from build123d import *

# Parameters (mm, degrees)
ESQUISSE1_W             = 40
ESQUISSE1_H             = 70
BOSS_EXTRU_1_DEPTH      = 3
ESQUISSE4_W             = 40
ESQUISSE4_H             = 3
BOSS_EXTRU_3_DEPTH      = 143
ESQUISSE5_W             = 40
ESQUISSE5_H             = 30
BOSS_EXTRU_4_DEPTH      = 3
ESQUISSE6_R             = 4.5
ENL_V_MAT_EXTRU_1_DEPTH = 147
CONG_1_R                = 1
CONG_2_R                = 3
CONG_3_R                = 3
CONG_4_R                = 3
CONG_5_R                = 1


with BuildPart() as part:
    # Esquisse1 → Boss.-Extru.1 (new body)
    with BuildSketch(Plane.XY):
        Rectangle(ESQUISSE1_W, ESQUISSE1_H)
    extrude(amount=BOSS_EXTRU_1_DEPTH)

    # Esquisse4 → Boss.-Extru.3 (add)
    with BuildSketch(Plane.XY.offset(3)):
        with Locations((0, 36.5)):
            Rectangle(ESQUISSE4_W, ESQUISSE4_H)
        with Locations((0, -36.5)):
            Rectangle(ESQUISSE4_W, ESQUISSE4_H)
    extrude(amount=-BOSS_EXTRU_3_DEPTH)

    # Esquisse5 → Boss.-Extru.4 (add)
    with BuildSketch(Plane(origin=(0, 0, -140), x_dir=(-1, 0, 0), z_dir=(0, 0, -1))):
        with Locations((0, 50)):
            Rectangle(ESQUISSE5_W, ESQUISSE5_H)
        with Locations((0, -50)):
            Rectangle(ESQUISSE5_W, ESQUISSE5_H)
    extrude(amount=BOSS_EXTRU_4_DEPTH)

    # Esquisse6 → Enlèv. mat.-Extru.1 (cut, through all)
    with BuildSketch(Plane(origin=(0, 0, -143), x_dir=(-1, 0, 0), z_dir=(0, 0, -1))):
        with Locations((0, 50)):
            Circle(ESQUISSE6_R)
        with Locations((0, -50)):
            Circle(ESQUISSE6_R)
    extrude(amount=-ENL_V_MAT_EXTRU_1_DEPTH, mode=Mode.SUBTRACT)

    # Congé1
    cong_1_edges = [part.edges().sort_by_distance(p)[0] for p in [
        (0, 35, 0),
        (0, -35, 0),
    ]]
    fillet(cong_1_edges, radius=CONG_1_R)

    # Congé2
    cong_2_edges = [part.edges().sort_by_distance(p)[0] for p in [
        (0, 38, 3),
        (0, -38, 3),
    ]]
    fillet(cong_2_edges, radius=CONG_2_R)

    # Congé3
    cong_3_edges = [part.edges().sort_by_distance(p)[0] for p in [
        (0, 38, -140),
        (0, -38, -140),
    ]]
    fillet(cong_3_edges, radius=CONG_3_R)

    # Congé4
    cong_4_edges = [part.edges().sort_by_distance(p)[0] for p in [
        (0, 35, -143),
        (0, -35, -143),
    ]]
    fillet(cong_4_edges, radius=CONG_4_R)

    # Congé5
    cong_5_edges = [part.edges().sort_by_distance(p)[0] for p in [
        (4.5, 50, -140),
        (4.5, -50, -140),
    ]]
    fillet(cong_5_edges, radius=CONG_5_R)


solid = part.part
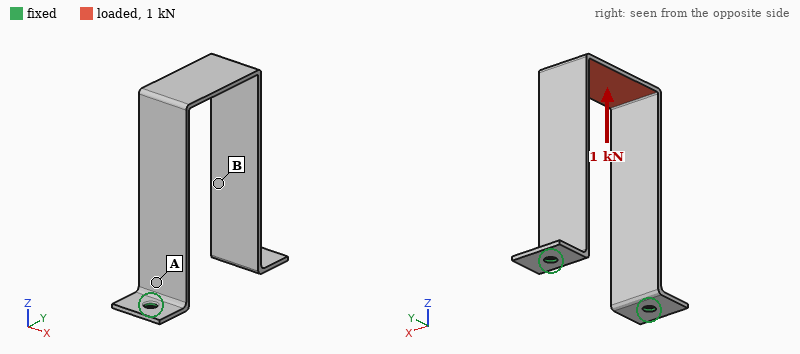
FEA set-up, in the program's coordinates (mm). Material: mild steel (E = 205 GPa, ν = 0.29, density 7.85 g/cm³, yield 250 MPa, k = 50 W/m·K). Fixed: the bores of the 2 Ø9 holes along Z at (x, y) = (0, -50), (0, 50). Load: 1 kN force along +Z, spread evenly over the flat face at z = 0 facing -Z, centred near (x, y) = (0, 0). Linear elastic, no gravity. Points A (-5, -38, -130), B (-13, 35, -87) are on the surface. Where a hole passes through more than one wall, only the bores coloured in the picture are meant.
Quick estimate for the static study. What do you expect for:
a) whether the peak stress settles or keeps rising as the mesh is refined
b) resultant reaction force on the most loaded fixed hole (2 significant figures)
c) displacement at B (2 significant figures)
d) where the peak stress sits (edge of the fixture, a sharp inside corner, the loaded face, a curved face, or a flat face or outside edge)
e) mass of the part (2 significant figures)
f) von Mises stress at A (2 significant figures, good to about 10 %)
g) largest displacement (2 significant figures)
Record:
keeps rising
500 N
0.057 mm
edge of the fixture
390 g
32 MPa
0.18 mm
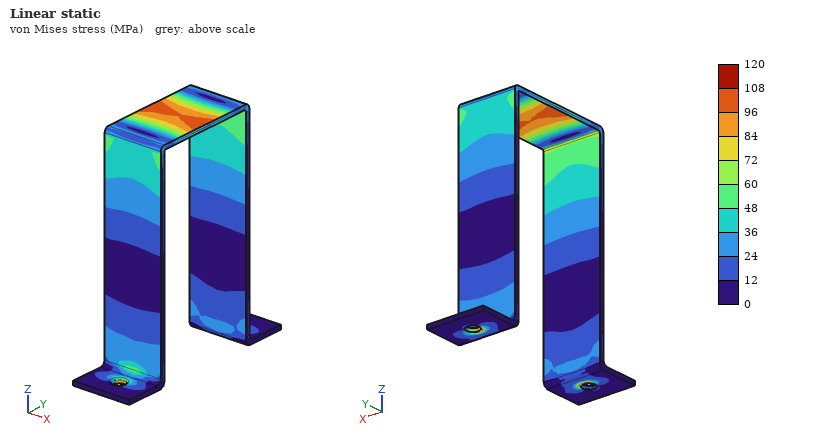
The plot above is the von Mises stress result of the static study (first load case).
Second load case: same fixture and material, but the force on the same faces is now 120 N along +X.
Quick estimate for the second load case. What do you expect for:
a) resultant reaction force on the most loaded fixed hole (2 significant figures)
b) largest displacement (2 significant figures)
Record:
60 N
0.37 mm
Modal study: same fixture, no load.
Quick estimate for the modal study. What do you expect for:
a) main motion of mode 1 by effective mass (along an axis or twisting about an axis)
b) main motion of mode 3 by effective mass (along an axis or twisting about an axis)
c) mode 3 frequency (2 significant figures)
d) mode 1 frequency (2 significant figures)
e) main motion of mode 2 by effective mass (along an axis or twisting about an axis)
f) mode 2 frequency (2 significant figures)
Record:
along Y
twisting about Z
360 Hz
130 Hz
along X
230 Hz
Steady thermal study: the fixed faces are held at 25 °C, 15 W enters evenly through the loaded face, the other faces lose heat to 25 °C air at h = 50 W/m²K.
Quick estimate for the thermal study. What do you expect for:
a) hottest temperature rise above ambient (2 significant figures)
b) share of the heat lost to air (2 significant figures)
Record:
41 K
98 %
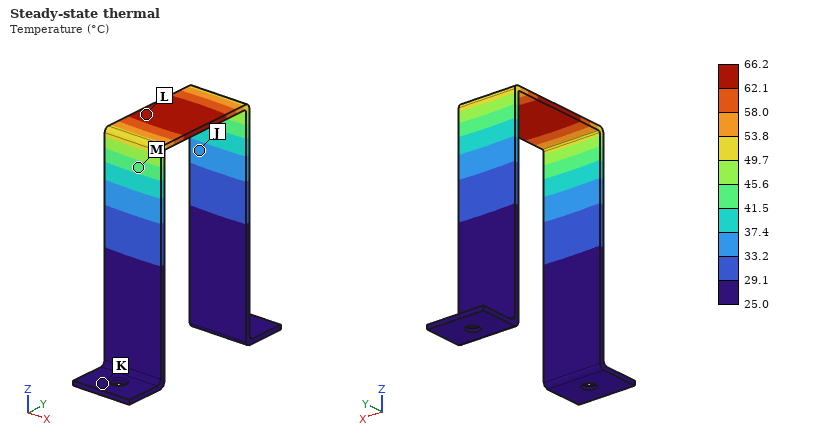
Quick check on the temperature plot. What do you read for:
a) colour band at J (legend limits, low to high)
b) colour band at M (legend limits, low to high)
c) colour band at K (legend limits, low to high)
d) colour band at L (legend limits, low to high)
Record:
33.2 to 37.4 °C
41.5 to 45.6 °C
25.0 to 29.1 °C
62.1 to 66.2 °C
